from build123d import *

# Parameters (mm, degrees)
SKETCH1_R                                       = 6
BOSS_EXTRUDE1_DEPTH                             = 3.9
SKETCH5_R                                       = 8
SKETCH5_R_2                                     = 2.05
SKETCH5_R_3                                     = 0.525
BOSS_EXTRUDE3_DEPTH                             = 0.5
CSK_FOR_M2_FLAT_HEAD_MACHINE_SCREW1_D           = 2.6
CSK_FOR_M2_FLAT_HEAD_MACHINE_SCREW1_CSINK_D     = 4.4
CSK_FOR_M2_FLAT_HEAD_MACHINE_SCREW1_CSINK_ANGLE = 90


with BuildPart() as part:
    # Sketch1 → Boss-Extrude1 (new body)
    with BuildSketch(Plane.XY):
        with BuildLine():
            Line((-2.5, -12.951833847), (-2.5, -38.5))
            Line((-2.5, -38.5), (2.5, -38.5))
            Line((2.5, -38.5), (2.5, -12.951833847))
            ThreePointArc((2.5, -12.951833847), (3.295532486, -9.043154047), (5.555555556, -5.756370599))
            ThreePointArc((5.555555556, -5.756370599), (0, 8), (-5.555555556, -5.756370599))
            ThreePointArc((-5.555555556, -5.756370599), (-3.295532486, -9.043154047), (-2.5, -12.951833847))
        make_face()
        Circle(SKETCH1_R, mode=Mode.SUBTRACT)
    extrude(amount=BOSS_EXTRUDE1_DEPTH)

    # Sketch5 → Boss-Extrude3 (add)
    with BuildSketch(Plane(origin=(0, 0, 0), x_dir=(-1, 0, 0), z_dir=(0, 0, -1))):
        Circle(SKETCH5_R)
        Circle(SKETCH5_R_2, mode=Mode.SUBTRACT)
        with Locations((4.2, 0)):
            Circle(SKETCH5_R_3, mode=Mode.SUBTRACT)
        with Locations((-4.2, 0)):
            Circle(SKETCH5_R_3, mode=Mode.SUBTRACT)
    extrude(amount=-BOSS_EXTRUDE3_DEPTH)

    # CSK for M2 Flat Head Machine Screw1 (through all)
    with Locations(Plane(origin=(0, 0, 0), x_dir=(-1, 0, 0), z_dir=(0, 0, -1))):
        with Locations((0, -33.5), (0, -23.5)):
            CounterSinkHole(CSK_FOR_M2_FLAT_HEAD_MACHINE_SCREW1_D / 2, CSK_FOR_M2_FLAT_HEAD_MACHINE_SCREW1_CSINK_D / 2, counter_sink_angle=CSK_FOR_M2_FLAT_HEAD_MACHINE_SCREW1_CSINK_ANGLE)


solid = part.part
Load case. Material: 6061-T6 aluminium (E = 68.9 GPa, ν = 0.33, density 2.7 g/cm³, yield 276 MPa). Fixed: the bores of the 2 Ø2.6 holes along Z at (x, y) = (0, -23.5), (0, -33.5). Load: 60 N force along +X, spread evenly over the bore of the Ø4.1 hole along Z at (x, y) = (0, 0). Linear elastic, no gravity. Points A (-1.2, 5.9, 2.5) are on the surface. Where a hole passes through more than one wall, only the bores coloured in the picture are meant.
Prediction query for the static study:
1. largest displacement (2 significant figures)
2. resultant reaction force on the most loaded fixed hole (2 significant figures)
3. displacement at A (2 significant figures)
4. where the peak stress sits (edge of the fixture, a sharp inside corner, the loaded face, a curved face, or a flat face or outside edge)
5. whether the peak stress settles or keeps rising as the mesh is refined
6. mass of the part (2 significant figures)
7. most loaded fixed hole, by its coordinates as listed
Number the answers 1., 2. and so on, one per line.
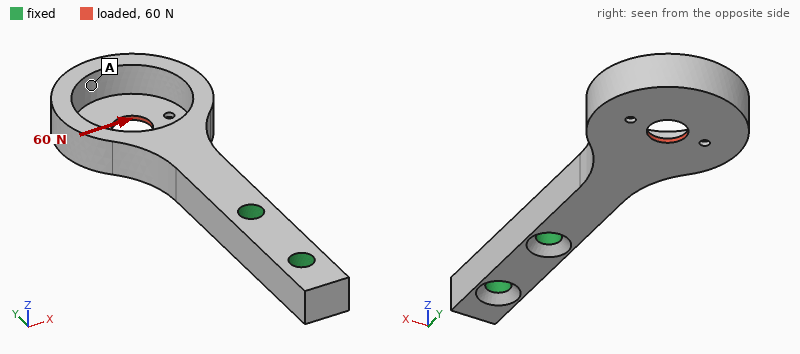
1. 0.15 mm
2. 89 N
3. 0.13 mm
4. edge of the fixture
5. keeps rising
6. 2.6 g
7. (0, -23.5)
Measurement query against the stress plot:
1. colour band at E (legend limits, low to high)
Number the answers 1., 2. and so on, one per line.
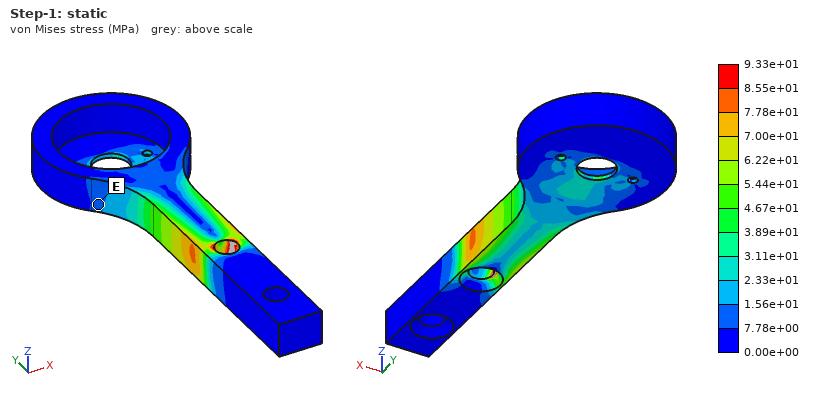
1. 7.78e+00 to 1.56e+01 MPa
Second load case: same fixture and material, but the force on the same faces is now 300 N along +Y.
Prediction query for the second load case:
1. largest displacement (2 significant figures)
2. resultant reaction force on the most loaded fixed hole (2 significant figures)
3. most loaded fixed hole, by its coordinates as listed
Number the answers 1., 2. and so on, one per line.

1. 0.13 mm
2. 290 N
3. (0, -23.5)
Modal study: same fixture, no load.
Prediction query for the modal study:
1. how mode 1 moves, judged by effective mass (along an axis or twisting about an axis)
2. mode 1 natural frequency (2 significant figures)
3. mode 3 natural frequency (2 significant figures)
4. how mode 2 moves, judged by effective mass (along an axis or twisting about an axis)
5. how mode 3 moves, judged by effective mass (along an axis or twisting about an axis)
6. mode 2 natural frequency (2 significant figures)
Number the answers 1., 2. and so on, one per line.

1. along Z
2. 2800 Hz
3. 8300 Hz
4. along X
5. twisting about Y
6. 3400 Hz
